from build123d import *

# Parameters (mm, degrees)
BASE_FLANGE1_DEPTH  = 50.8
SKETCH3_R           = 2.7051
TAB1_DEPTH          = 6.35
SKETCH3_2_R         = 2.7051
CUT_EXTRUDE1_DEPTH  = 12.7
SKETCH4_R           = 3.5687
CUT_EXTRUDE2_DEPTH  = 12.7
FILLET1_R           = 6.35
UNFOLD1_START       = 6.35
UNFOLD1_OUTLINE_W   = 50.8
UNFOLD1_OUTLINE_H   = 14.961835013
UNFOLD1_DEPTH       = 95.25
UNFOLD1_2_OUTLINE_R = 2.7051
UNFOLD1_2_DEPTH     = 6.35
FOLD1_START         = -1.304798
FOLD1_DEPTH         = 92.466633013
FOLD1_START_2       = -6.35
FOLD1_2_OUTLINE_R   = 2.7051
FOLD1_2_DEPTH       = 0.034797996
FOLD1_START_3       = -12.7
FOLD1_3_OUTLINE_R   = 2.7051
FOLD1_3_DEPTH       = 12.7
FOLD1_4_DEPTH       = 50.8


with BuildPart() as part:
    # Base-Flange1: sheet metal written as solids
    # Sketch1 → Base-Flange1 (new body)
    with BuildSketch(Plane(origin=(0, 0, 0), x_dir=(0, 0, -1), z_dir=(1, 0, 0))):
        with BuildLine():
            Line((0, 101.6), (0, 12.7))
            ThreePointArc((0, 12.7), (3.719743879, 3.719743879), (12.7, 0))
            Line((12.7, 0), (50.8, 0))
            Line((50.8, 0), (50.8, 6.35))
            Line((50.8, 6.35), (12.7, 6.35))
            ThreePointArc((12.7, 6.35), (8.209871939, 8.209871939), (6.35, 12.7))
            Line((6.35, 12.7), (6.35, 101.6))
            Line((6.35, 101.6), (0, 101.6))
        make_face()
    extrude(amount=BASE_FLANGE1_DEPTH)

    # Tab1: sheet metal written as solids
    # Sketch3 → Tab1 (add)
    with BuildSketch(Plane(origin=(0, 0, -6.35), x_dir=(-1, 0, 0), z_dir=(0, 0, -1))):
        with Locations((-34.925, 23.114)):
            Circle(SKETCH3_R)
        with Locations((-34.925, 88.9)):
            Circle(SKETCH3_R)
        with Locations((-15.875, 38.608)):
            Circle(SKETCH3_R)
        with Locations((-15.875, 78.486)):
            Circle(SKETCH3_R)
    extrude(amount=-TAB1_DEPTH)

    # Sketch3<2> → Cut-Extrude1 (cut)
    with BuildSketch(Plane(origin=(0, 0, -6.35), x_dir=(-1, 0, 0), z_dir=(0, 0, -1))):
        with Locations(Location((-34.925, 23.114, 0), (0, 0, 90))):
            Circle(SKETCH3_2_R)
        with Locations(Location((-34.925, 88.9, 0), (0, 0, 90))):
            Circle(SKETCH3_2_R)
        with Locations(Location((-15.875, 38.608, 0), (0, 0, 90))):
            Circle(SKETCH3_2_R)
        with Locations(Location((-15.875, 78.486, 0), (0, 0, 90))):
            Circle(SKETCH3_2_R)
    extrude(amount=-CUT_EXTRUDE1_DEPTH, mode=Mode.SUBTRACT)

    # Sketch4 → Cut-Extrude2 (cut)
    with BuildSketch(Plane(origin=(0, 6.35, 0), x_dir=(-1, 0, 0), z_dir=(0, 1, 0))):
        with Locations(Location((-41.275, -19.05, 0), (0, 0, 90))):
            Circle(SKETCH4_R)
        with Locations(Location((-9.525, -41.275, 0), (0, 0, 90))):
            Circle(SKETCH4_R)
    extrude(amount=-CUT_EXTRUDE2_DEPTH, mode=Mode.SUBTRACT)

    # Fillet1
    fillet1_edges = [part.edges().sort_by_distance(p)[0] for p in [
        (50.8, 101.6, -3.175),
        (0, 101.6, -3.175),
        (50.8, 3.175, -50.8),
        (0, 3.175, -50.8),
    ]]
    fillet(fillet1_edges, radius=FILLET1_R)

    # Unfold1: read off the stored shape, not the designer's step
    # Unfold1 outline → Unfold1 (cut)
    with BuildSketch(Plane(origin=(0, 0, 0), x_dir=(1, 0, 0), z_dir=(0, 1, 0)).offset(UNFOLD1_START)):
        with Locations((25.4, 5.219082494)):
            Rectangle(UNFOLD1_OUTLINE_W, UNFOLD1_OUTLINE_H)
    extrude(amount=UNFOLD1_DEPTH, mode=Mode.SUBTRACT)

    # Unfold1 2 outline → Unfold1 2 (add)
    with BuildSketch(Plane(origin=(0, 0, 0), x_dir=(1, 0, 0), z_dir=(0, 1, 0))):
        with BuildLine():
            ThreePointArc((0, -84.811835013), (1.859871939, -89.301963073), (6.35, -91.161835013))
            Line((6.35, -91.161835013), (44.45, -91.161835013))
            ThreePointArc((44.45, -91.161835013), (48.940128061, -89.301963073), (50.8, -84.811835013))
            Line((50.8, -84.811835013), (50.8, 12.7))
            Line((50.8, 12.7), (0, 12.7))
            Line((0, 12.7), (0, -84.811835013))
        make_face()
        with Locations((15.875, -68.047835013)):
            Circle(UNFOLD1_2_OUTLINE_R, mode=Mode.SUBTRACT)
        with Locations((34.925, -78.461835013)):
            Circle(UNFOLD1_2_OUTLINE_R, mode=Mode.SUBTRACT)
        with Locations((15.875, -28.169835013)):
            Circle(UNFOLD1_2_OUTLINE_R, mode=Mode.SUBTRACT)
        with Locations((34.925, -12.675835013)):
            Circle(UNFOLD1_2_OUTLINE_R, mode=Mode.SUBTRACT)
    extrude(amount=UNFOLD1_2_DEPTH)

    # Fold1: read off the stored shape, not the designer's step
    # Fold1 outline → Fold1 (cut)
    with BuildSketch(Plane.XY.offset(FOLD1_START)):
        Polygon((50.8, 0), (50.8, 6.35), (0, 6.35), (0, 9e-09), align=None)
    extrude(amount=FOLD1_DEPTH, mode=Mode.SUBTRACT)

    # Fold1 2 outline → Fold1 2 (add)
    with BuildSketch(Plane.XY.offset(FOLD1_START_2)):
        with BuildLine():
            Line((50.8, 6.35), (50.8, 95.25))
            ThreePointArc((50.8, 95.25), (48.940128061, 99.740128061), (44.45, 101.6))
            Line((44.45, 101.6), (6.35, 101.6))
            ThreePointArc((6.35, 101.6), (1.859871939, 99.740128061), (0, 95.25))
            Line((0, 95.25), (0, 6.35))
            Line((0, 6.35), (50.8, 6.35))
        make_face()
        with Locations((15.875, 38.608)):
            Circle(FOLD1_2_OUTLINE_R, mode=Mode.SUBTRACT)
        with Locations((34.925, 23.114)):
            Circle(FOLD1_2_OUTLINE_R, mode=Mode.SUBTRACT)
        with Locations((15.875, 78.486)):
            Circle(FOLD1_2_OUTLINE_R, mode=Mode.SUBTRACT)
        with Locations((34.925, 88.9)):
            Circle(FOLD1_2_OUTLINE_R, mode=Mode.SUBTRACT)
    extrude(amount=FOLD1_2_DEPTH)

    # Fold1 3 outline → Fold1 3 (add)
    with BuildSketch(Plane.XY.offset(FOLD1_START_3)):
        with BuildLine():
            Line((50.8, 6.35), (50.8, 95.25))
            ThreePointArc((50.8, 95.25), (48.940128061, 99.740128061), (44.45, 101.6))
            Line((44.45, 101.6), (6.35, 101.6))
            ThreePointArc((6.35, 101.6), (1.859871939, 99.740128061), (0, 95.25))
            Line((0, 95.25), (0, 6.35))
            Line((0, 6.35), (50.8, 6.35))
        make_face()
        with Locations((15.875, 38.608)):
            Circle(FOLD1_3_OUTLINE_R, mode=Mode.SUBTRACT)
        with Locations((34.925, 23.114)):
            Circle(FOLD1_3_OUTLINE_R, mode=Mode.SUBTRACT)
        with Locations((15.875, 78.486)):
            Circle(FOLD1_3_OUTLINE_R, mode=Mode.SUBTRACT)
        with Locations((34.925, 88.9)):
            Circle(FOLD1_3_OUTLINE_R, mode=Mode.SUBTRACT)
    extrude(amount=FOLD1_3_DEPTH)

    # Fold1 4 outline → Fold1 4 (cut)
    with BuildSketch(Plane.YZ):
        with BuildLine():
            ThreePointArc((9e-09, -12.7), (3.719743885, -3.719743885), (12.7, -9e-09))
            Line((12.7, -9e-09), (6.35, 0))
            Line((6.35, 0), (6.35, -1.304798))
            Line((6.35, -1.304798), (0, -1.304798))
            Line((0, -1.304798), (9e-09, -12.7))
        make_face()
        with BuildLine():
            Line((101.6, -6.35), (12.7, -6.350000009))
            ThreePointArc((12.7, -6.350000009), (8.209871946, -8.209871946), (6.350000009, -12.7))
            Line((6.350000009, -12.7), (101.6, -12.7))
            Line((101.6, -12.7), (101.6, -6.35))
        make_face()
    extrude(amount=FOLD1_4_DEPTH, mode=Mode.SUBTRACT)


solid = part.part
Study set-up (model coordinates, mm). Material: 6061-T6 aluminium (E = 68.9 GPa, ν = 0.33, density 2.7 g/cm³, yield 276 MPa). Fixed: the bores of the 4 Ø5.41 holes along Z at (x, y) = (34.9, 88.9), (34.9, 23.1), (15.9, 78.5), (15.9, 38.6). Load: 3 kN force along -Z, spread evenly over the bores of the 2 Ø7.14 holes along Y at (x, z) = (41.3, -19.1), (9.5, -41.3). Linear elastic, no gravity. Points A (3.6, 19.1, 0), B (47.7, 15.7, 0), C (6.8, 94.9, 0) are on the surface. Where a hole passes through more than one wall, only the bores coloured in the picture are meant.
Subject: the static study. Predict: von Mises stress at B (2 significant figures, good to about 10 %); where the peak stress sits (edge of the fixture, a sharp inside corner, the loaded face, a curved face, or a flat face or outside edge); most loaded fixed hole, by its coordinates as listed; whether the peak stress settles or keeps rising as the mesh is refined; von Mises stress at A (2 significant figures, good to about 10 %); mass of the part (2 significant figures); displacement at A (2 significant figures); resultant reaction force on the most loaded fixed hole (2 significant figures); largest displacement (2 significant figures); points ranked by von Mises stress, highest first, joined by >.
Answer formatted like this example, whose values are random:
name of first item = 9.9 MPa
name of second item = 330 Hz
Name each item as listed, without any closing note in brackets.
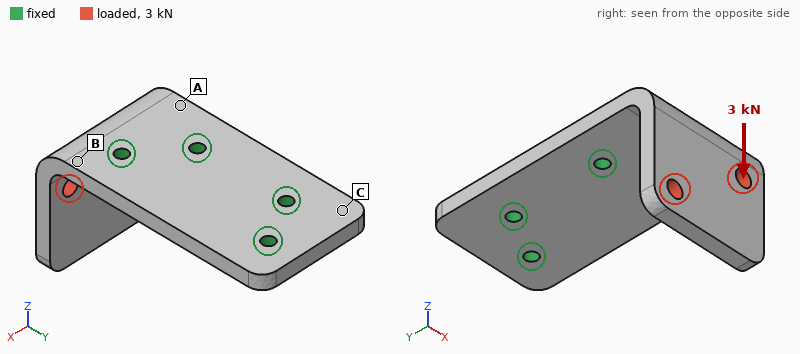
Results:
von Mises stress at B = 95 MPa
where the peak stress sits = edge of the fixture
most loaded fixed hole, by its coordinates as listed = (34.9, 23.1)
whether the peak stress settles or keeps rising as the mesh is refined = keeps rising
von Mises stress at A = 74 MPa
mass of the part = 120 g
displacement at A = 0.11 mm
resultant reaction force on the most loaded fixed hole = 3.0 kN
largest displacement = 0.64 mm
points ranked by von Mises stress, highest first, joined by > = B > A > C
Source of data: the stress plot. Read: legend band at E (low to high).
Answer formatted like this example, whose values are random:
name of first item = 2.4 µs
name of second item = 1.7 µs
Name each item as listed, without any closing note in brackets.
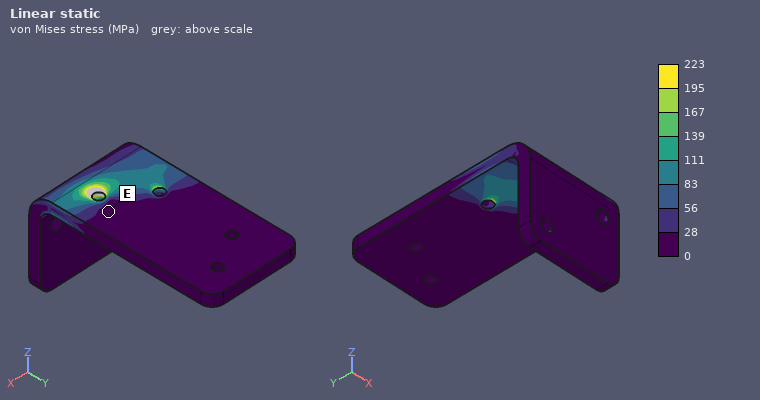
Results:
legend band at E = 0 to 28 MPa
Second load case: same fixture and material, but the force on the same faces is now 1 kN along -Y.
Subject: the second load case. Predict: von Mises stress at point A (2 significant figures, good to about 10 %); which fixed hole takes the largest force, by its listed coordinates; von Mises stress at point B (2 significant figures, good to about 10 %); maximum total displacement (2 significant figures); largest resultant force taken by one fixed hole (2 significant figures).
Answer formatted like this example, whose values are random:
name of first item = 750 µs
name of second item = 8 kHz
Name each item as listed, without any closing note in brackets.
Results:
von Mises stress at point A = 58 MPa
which fixed hole takes the largest force, by its listed coordinates = (34.9, 23.1)
von Mises stress at point B = 65 MPa
maximum total displacement = 0.57 mm
largest resultant force taken by one fixed hole = 690 N
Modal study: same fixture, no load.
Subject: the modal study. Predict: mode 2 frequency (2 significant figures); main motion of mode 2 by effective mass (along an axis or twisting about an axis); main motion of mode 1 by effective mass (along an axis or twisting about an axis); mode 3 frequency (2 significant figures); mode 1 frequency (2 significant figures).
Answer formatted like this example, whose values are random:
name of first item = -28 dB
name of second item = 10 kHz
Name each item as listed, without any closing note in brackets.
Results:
mode 2 frequency = 2100 Hz
main motion of mode 2 by effective mass = along X
main motion of mode 1 by effective mass = along Y
mode 3 frequency = 4600 Hz
mode 1 frequency = 1400 Hz
